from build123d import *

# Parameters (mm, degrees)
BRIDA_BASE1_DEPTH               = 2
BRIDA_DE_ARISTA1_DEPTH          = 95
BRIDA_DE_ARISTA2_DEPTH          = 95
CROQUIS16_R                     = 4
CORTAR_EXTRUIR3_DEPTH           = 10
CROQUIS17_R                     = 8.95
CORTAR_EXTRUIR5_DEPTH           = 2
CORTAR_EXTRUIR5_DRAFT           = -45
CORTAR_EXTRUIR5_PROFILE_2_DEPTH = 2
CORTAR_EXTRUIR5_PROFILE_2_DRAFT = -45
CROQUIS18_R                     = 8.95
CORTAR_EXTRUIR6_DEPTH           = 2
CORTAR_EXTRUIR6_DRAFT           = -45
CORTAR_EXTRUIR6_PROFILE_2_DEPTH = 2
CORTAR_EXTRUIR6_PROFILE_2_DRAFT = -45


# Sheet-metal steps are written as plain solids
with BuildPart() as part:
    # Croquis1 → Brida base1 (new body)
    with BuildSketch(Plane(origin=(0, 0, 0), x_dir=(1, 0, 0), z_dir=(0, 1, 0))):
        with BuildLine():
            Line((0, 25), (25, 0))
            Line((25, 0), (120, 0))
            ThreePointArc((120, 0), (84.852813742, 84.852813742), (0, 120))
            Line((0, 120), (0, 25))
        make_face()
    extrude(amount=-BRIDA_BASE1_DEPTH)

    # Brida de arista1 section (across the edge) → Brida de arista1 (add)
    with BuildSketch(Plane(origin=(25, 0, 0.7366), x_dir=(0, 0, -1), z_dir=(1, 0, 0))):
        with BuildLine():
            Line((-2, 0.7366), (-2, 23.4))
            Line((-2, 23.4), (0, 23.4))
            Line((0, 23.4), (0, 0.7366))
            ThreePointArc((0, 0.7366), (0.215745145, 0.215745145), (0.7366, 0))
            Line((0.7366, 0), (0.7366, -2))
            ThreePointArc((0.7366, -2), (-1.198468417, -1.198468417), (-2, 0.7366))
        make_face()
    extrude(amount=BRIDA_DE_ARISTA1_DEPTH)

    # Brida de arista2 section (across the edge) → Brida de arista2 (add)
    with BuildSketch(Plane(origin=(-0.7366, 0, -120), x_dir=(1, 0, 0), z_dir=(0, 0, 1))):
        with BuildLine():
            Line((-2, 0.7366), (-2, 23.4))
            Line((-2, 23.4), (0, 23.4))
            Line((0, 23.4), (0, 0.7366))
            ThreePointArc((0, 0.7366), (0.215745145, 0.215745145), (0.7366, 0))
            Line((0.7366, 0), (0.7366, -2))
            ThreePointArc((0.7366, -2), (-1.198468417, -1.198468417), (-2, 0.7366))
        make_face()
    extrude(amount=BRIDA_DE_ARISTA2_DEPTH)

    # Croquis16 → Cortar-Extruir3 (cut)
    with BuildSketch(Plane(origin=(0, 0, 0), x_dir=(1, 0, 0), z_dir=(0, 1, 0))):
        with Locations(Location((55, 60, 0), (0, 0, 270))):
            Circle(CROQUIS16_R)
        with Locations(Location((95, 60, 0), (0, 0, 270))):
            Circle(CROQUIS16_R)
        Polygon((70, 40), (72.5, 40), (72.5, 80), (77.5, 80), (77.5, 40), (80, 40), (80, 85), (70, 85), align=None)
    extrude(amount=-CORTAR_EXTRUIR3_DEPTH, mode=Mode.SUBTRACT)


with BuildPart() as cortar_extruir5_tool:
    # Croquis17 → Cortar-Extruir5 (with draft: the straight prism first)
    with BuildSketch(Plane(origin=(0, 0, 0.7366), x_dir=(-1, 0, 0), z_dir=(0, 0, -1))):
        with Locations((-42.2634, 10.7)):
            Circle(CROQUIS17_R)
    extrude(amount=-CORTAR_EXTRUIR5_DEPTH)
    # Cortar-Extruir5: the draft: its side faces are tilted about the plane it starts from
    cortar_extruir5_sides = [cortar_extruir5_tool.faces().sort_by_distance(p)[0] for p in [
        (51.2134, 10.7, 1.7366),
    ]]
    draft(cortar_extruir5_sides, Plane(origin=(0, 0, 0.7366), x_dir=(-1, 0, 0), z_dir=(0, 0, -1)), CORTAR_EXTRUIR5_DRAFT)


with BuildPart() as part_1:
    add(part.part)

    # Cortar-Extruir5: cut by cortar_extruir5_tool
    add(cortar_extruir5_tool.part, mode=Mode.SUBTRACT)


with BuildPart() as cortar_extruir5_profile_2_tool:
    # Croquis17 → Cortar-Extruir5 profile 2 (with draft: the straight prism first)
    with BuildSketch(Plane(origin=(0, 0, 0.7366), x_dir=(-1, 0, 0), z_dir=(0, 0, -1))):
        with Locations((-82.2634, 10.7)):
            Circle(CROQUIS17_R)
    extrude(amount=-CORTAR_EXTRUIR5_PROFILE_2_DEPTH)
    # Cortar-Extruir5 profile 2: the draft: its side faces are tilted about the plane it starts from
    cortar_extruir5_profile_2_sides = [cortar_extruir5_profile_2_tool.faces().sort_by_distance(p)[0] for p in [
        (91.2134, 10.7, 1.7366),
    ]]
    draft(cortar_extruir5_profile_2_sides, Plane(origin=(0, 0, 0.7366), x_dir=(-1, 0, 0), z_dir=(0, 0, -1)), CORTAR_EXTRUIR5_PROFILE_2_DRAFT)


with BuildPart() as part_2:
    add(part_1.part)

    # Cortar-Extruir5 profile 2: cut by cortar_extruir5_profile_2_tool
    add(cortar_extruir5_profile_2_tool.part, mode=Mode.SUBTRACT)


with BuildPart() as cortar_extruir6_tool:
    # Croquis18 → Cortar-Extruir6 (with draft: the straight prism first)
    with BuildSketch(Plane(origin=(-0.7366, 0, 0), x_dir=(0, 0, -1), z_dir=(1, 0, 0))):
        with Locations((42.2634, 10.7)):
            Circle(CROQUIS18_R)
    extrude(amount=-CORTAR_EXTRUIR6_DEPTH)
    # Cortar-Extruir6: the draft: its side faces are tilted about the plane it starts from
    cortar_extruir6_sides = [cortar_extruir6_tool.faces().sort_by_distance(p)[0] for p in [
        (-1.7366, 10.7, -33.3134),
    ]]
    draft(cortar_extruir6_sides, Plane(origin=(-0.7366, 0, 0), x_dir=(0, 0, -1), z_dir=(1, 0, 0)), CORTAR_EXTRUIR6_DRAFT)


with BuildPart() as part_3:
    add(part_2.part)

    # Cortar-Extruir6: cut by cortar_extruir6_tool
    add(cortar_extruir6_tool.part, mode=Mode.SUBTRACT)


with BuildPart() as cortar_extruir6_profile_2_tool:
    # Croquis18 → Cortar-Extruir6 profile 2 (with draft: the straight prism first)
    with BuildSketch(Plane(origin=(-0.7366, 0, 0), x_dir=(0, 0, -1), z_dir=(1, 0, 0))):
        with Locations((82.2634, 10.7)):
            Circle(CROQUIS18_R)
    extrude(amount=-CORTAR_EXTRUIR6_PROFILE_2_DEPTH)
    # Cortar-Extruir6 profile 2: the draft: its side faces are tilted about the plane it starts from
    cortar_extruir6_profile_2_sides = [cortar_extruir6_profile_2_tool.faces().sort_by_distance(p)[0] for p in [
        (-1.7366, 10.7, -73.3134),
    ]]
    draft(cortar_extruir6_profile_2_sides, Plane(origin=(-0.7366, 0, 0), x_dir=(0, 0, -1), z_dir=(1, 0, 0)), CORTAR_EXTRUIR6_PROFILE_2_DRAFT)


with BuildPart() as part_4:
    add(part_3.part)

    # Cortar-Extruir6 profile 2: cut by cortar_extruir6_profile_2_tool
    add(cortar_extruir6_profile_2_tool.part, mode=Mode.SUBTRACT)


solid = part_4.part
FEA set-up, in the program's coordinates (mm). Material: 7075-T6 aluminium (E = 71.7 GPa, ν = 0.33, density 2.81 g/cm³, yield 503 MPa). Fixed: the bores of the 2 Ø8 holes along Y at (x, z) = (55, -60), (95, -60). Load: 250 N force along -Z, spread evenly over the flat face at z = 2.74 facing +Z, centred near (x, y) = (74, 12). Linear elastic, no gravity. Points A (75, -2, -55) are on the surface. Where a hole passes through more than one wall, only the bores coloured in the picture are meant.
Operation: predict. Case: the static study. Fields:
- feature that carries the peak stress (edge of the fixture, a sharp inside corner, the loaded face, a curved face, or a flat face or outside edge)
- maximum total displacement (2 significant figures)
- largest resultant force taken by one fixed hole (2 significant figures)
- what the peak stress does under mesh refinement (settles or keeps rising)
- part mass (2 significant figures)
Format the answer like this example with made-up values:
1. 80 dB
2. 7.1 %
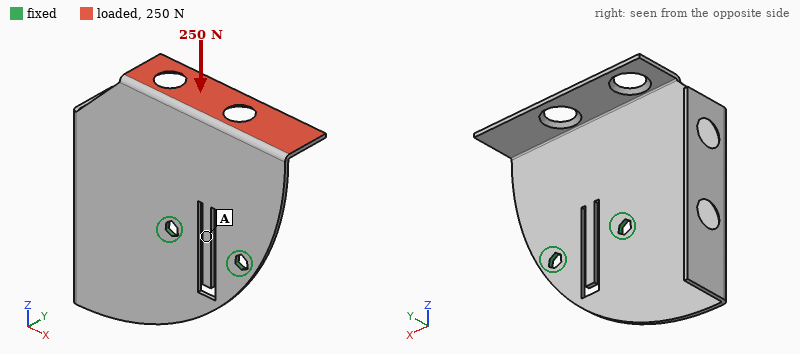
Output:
1. edge of the fixture
2. 1.8 mm
3. 130 N
4. keeps rising
5. 82 g
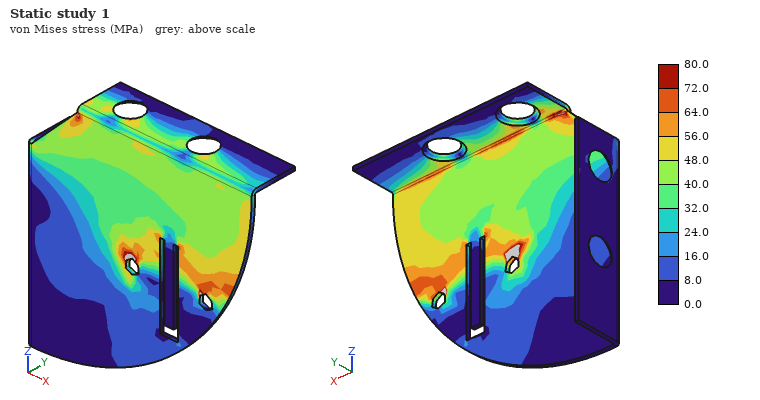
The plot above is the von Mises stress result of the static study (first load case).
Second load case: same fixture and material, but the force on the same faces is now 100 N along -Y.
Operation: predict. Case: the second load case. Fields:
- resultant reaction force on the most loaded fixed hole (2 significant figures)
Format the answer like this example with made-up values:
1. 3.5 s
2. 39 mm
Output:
1. 51 N
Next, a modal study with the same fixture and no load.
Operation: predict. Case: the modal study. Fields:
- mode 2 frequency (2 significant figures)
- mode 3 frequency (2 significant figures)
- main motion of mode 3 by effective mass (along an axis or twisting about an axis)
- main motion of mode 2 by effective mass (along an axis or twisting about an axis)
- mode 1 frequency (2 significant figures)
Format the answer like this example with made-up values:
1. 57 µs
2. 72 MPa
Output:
1. 300 Hz
2. 390 Hz
3. twisting about Z
4. along Y
5. 250 Hz
